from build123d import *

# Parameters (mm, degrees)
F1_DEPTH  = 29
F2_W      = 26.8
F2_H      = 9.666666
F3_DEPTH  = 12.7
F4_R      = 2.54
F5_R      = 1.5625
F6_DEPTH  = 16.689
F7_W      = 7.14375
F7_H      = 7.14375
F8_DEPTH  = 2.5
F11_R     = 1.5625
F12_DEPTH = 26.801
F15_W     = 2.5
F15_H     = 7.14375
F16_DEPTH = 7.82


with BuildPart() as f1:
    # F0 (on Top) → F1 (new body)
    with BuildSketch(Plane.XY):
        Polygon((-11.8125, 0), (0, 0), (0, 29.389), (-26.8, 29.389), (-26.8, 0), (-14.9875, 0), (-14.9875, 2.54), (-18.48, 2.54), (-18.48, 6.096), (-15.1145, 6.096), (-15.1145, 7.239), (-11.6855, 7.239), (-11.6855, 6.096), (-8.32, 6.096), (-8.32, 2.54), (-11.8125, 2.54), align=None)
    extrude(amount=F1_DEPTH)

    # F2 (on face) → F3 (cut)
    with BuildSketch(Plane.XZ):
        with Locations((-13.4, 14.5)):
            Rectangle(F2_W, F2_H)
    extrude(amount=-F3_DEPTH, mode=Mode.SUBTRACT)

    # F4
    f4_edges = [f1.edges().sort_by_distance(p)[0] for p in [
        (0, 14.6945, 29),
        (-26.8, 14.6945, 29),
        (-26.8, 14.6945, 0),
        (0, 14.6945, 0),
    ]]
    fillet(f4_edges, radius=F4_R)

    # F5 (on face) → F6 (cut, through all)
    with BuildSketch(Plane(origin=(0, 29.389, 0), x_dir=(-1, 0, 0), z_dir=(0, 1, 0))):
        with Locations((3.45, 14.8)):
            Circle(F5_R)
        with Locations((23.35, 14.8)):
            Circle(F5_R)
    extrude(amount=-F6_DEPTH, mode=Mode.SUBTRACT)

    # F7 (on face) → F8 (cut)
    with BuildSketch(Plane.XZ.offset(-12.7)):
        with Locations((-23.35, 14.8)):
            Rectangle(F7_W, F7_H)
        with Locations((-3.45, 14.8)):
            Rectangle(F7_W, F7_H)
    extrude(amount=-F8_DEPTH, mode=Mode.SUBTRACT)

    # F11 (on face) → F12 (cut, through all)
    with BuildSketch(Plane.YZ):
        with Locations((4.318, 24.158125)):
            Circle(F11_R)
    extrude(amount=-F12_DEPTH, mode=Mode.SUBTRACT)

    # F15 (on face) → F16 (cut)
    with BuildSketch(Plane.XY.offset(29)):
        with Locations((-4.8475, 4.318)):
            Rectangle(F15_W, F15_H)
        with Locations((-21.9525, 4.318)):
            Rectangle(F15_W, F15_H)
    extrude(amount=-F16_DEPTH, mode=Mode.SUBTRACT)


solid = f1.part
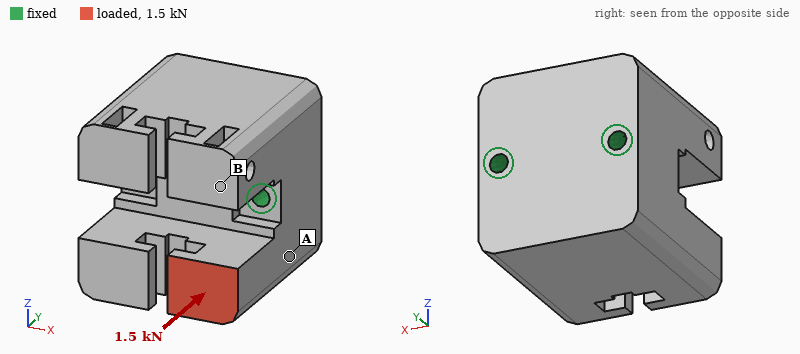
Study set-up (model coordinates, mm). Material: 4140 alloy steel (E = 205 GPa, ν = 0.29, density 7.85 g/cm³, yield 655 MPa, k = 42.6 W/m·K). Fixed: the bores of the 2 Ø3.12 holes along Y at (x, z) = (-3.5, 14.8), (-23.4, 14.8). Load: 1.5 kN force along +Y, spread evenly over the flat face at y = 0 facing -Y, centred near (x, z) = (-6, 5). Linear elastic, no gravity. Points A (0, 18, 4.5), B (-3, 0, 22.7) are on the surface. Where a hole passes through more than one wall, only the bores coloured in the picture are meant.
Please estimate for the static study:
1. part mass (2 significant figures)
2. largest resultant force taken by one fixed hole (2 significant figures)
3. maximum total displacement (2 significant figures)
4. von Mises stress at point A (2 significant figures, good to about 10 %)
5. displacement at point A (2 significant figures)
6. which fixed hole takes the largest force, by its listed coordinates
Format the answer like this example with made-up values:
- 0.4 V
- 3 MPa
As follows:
- 140 g
- 1.2 kN
- 8.0 µm
- 14 MPa
- 1.8 µm
- (-3.5, 14.8)
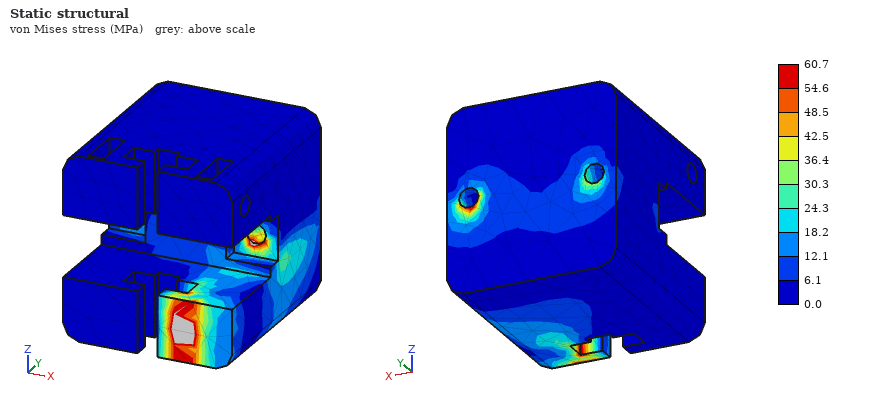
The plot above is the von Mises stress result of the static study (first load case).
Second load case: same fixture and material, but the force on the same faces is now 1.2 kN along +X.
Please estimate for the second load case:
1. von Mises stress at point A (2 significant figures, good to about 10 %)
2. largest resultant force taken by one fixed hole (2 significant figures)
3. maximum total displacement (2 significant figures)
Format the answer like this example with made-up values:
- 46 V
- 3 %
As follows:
- 25 MPa
- 1.4 kN
- 14 µm
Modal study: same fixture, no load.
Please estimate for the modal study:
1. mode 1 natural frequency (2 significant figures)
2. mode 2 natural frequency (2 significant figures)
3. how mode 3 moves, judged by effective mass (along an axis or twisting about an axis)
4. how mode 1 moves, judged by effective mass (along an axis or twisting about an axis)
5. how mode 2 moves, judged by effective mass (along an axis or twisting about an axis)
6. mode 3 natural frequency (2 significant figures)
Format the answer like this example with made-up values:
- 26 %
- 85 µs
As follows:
- 14 kHz
- 19 kHz
- along X
- along Z
- along Y
- 21 kHz
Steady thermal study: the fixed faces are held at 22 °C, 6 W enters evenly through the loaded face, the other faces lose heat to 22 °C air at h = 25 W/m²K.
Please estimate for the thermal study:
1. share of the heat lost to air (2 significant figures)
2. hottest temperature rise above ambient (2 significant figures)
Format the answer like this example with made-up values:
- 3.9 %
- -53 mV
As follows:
- 7.1 %
- 31 K
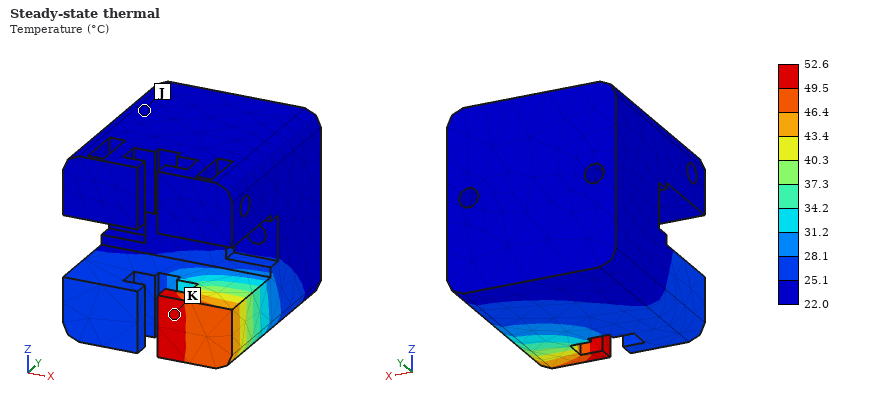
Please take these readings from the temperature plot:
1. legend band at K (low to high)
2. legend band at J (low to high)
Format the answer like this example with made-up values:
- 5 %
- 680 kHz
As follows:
- 49.5 to 52.6 °C
- 22.0 to 25.1 °C
